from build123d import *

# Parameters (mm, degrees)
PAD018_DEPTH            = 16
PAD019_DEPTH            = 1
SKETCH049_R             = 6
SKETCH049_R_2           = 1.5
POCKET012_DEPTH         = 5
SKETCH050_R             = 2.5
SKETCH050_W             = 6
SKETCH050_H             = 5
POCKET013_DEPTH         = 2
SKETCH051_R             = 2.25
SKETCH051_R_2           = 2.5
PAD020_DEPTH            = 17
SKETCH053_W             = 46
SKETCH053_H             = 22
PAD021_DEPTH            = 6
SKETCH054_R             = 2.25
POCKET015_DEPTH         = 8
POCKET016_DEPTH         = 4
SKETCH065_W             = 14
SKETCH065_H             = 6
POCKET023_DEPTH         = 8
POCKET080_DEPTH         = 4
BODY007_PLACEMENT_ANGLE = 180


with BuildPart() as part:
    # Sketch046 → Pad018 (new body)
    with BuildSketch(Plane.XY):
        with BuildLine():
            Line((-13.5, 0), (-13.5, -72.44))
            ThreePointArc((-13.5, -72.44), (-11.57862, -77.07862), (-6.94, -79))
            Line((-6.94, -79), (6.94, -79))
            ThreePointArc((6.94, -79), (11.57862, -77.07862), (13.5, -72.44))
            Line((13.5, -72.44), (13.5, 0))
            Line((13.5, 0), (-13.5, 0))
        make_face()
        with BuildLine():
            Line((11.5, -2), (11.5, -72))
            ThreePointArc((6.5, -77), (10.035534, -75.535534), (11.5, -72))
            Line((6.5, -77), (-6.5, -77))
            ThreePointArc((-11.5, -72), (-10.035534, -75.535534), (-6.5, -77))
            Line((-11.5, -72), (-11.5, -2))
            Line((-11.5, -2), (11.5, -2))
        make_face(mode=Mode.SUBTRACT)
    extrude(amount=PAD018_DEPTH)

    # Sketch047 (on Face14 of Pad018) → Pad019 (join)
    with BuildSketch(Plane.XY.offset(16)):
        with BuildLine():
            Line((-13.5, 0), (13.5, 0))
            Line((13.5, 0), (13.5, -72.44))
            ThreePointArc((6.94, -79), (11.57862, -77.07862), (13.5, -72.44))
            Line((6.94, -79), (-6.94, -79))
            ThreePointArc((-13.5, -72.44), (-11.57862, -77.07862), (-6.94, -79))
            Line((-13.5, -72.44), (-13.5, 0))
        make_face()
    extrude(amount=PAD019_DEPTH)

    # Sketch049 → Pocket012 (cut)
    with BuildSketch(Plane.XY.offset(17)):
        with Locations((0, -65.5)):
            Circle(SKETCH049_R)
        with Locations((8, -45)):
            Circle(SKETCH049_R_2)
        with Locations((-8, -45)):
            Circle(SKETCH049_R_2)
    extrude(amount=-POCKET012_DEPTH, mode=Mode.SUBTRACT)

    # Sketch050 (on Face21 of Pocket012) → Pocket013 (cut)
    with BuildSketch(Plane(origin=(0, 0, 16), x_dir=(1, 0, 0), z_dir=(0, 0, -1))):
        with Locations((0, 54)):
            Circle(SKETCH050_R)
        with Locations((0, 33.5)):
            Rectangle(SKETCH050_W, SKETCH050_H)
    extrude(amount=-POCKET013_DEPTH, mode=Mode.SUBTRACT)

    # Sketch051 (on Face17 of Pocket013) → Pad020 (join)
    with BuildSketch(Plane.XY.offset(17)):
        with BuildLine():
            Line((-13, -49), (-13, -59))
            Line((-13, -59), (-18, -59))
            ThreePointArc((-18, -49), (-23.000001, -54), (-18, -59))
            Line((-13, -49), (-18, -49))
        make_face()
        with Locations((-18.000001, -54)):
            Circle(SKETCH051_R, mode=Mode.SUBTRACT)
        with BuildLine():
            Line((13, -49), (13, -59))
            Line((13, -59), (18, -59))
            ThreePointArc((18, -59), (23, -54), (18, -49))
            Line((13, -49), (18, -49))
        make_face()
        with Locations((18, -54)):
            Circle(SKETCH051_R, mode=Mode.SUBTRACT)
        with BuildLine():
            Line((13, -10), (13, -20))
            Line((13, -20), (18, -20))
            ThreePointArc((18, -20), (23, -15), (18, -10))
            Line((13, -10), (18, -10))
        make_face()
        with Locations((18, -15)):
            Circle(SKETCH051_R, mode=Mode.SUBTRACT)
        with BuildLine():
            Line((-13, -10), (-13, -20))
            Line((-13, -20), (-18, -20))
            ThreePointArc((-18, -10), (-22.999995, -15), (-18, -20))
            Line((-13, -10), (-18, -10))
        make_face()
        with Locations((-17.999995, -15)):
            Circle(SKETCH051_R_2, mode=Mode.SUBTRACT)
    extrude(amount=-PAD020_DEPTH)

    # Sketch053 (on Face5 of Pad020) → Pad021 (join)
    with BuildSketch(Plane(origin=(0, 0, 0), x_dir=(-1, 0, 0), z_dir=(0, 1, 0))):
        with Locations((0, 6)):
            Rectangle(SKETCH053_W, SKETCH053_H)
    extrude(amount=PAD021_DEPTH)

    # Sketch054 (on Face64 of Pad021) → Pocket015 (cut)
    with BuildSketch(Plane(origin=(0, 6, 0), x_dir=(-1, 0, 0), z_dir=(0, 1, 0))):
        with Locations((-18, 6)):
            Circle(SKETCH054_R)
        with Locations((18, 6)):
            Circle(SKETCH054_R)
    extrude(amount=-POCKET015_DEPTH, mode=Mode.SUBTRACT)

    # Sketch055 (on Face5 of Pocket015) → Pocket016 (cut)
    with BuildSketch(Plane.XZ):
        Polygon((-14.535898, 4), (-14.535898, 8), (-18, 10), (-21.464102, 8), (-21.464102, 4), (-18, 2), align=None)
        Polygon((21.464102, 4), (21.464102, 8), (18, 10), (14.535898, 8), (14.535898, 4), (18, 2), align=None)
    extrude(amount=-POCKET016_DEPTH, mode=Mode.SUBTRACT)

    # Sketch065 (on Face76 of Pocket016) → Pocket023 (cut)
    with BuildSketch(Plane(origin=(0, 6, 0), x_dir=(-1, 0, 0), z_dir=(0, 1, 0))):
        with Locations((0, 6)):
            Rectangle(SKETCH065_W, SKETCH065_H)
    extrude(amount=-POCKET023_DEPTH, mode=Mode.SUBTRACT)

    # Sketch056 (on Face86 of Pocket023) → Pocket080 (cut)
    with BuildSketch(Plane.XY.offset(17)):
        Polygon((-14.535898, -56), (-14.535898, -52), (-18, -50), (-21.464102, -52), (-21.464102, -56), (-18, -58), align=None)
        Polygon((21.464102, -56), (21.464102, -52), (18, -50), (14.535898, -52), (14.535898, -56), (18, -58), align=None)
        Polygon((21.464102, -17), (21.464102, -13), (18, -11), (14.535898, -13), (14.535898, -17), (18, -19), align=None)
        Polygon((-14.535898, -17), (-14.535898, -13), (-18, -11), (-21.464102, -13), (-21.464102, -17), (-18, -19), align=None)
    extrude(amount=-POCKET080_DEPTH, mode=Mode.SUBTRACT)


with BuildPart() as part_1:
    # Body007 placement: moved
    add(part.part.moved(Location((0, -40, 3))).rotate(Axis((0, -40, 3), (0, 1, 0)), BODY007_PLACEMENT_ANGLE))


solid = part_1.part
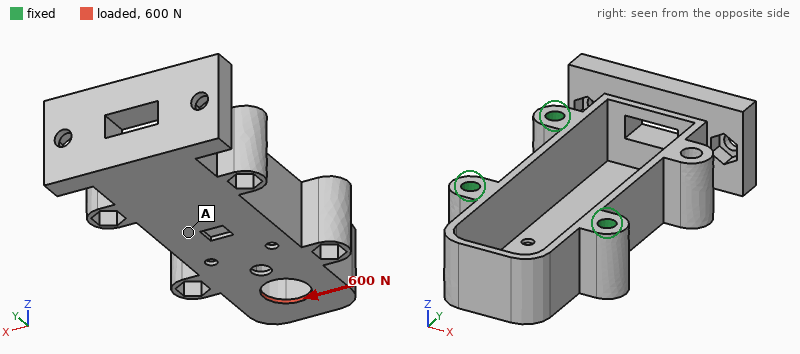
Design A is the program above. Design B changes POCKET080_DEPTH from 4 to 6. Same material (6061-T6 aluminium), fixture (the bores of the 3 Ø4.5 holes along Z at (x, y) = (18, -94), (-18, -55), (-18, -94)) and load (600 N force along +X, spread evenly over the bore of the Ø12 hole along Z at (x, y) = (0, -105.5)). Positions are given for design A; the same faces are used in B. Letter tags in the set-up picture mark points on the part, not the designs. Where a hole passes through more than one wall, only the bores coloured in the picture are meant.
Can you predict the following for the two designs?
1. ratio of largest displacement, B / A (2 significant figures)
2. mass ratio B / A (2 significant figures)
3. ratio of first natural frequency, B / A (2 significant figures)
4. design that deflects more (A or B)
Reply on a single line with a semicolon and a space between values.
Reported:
1.1; 0.99; 0.99; B
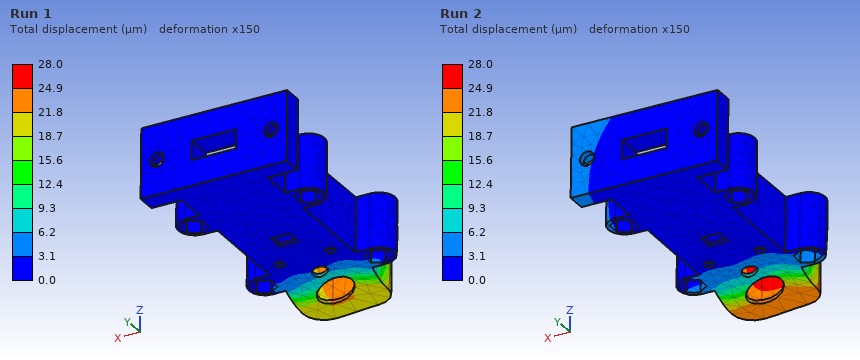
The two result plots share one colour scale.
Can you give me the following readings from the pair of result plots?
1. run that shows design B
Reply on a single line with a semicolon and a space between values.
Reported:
Run 2
